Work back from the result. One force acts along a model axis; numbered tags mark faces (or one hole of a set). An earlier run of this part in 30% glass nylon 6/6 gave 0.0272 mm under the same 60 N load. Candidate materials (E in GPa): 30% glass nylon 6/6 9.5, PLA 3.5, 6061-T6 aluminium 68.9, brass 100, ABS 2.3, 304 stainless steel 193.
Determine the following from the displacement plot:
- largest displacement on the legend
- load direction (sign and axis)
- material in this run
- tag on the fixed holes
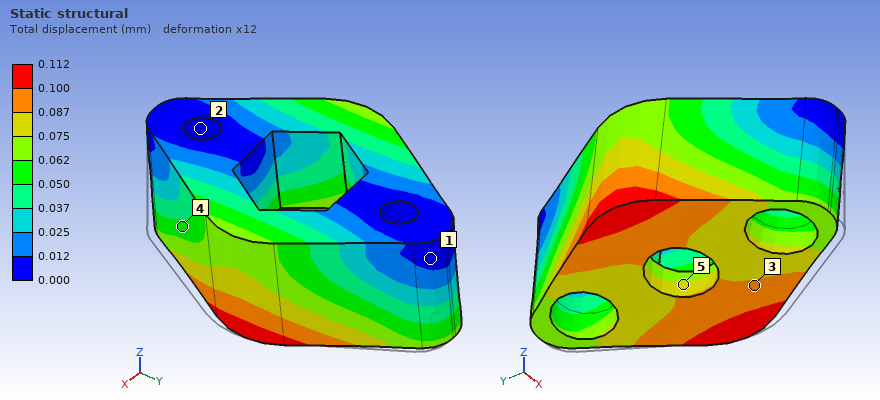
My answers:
0.112 mm
-X
ABS
2
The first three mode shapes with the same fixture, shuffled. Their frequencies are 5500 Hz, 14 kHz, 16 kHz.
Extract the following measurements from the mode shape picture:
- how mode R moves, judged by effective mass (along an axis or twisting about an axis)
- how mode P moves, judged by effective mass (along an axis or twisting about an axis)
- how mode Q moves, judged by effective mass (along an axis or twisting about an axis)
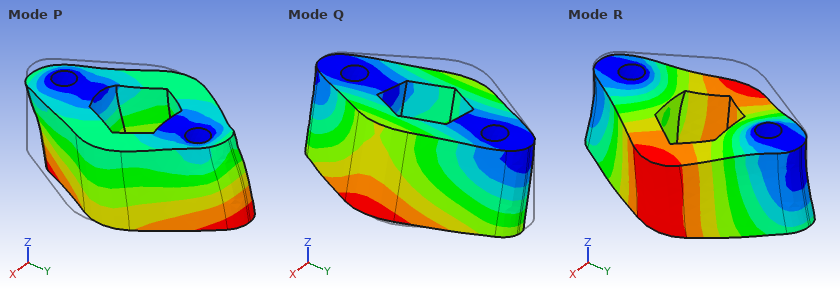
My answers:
along Z
along Y
along X
